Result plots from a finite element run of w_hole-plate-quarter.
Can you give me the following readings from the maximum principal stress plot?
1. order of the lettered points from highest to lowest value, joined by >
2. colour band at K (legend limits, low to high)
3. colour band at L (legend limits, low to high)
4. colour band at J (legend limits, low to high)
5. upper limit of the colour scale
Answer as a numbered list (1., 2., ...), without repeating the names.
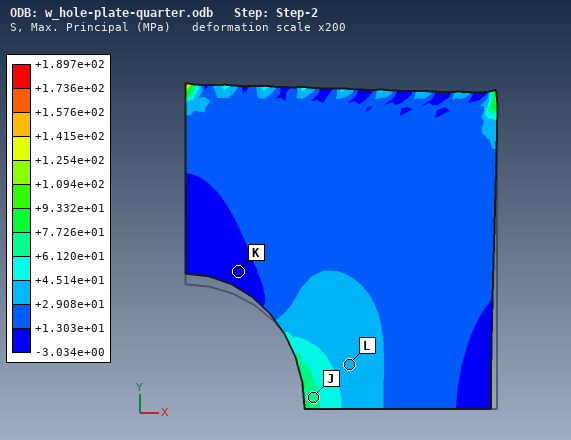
1. J > L > K
2. -3.034e+00 to +1.303e+01 MPa
3. +2.908e+01 to +4.514e+01 MPa
4. +6.120e+01 to +7.726e+01 MPa
5. +1.897e+02 MPa
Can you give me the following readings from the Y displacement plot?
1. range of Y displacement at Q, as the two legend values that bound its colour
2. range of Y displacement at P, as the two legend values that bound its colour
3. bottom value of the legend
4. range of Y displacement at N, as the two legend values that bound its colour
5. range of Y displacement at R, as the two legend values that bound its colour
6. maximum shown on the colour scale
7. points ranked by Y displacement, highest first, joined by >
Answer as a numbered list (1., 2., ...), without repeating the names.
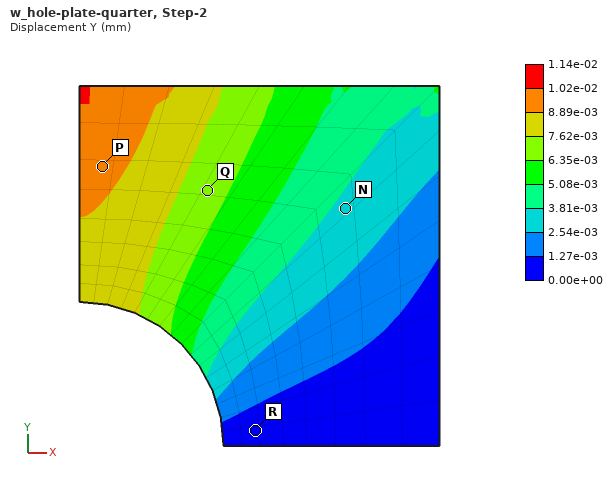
1. 6.35e-03 to 7.62e-03 mm
2. 8.89e-03 to 1.02e-02 mm
3. 0.00e+00 mm
4. 2.54e-03 to 3.81e-03 mm
5. 0.00e+00 to 1.27e-03 mm
6. 1.14e-02 mm
7. P > Q > N > R
